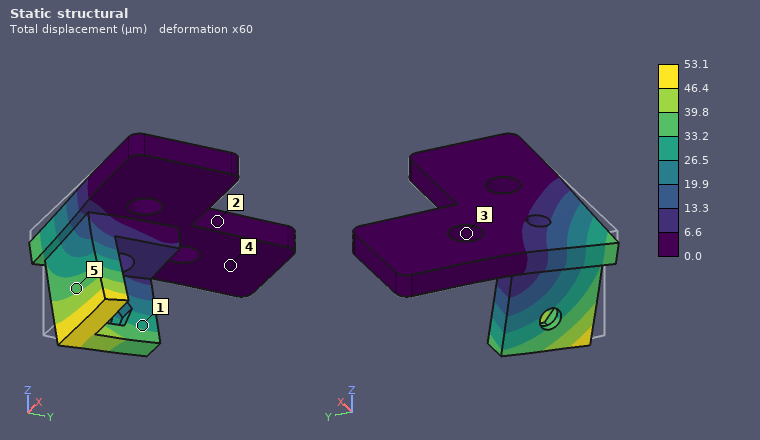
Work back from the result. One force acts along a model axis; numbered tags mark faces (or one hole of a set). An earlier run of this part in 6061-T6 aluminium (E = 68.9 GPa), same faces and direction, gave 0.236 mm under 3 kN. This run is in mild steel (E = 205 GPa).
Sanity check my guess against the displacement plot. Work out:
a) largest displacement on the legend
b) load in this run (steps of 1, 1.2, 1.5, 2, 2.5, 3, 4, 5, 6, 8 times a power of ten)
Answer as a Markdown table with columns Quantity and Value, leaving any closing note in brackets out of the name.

| Quantity | Value |
|---|---|
| largest displacement on the legend | 53.1 µm |
| load in this run | 2 kN |
